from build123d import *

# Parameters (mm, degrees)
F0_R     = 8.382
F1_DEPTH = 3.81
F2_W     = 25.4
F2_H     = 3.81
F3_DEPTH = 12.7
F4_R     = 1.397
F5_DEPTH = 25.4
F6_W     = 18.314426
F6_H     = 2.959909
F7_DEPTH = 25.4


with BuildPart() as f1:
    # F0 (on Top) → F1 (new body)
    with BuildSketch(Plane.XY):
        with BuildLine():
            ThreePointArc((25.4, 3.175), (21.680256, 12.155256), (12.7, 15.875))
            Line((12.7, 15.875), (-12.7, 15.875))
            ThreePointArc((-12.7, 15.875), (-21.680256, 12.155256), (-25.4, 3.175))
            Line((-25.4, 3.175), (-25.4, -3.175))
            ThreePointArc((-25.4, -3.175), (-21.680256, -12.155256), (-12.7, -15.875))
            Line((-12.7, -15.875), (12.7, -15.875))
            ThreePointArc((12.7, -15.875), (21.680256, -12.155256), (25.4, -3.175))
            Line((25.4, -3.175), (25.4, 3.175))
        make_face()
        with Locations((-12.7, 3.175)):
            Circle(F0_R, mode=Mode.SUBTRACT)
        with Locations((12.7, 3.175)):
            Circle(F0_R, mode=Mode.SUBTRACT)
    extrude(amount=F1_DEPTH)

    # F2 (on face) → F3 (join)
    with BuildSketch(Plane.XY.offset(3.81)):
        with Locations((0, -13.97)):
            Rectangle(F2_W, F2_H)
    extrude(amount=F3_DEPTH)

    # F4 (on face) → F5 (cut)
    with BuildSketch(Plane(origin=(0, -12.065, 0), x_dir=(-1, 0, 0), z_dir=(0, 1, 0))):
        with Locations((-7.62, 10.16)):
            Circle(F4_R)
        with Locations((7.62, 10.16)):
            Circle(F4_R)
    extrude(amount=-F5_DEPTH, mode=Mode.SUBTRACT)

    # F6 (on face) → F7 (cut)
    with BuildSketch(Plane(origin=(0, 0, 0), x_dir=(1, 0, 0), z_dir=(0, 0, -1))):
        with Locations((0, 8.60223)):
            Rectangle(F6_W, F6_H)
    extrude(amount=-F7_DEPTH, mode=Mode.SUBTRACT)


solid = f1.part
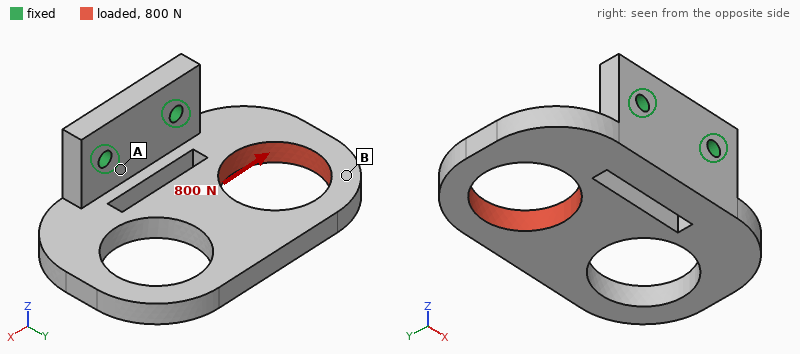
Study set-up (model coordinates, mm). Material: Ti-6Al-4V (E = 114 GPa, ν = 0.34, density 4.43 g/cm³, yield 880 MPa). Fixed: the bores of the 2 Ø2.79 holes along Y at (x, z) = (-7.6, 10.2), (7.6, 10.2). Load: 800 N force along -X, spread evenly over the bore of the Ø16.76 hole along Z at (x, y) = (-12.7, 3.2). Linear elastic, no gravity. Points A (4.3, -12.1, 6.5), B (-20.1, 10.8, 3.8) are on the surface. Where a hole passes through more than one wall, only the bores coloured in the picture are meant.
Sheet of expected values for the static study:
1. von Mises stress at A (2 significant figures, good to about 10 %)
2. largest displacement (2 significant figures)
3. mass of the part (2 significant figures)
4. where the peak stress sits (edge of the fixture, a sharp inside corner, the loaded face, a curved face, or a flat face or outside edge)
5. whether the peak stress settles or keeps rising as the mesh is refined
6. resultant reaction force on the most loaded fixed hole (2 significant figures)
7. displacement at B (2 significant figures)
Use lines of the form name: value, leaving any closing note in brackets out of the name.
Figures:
von Mises stress at A: 76 MPa
largest displacement: 0.11 mm
mass of the part: 22 g
where the peak stress sits: edge of the fixture
whether the peak stress settles or keeps rising as the mesh is refined: keeps rising
resultant reaction force on the most loaded fixed hole: 900 N
displacement at B: 0.10 mm
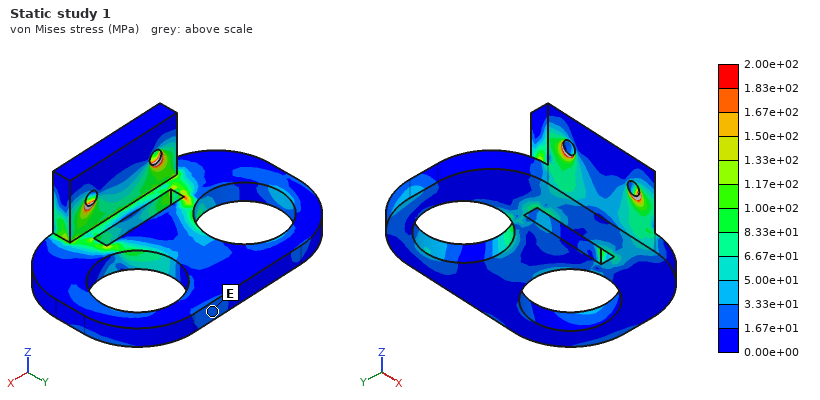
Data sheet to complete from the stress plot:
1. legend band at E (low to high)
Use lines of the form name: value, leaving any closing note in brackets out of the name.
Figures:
legend band at E: 1.67e+01 to 3.33e+01 MPa
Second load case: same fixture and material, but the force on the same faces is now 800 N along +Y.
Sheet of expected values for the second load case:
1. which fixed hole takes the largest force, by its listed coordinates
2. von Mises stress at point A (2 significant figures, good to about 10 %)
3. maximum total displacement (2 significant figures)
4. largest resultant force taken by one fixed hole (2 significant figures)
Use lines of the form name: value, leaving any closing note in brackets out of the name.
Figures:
which fixed hole takes the largest force, by its listed coordinates: (-7.6, 10.2)
von Mises stress at point A: 43 MPa
maximum total displacement: 0.12 mm
largest resultant force taken by one fixed hole: 930 N
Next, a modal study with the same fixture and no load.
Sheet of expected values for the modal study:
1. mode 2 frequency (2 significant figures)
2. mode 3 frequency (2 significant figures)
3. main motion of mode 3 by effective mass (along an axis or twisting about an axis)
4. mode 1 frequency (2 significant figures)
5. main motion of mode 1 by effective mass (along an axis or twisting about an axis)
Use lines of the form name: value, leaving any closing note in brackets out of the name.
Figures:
mode 2 frequency: 3600 Hz
mode 3 frequency: 4800 Hz
main motion of mode 3 by effective mass: along X
mode 1 frequency: 1900 Hz
main motion of mode 1 by effective mass: along Z
